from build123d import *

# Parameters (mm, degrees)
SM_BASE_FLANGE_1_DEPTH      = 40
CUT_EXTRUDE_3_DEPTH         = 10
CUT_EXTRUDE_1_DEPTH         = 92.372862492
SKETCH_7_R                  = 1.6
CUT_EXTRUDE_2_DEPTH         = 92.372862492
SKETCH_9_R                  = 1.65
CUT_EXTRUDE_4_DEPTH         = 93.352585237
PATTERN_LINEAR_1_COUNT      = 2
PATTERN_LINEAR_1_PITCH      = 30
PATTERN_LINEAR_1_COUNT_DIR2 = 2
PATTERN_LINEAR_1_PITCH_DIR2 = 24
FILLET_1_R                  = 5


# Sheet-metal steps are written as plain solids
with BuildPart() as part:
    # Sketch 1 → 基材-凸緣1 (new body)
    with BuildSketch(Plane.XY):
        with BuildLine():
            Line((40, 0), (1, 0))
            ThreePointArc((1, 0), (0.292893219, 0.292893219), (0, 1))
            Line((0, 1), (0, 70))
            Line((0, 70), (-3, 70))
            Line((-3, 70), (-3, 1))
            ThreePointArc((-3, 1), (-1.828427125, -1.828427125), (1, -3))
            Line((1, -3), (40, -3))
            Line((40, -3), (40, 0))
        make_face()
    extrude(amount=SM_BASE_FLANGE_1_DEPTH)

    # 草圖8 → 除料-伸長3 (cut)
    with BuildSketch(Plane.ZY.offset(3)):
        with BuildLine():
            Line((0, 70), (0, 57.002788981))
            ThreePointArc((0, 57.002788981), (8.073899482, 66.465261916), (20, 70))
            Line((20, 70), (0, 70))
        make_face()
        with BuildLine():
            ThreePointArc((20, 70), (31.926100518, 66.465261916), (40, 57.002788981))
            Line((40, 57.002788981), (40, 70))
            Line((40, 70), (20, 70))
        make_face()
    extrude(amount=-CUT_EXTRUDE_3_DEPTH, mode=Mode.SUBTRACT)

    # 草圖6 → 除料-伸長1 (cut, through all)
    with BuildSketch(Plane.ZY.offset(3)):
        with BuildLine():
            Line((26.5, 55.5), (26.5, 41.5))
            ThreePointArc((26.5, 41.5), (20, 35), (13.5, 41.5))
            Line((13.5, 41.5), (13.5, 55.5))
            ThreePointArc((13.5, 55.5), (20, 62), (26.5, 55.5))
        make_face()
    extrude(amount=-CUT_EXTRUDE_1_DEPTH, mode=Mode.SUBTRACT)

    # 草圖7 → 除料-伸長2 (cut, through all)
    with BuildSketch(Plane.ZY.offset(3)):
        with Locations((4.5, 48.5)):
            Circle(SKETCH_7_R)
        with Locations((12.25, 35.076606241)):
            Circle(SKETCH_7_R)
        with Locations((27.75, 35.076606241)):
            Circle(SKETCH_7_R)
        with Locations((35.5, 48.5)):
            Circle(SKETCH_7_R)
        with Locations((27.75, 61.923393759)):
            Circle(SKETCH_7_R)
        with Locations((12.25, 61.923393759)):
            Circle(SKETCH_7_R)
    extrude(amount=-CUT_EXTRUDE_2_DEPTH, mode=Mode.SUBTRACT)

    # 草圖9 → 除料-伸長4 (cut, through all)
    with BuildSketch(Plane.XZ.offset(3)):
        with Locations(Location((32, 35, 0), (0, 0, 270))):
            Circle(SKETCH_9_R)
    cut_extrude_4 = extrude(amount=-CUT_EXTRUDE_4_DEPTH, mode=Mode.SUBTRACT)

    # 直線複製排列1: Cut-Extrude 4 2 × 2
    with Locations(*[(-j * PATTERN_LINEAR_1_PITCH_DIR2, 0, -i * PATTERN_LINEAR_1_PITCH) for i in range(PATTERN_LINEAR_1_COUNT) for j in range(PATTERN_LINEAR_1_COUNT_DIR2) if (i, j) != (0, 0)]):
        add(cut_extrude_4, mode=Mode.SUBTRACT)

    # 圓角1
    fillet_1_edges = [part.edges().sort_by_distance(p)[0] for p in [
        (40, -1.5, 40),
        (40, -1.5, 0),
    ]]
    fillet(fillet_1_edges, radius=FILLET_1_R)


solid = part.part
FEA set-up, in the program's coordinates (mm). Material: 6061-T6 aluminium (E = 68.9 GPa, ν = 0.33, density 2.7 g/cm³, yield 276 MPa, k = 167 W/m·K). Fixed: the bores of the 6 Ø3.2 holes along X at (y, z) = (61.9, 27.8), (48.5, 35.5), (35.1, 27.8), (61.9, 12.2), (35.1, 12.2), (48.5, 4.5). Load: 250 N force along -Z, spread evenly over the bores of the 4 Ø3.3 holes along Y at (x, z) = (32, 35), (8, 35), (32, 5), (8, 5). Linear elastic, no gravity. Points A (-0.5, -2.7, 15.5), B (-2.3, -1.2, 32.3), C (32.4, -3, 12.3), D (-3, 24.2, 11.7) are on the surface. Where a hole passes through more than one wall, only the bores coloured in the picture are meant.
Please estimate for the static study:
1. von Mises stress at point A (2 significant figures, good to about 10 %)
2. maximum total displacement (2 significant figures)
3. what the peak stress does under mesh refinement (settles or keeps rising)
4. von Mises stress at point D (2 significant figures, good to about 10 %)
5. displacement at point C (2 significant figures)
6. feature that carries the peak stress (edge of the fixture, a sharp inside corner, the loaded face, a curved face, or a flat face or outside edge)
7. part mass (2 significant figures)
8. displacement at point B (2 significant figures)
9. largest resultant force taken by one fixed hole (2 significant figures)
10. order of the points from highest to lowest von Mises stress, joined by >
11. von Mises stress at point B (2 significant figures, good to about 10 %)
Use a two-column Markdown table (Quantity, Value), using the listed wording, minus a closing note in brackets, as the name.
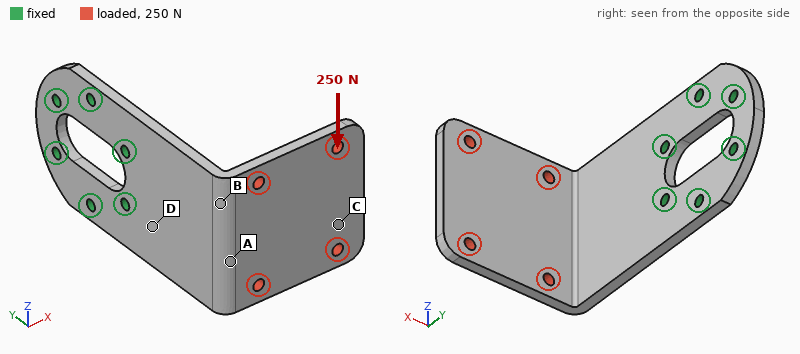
| Quantity | Value |
|---|---|
| von Mises stress at point A | 32 MPa |
| maximum total displacement | 0.68 mm |
| what the peak stress does under mesh refinement | keeps rising |
| von Mises stress at point D | 55 MPa |
| displacement at point C | 0.53 mm |
| feature that carries the peak stress | edge of the fixture |
| part mass | 32 g |
| displacement at point B | 0.18 mm |
| largest resultant force taken by one fixed hole | 380 N |
| order of the points from highest to lowest von Mises stress, joined by > | D > B > A > C |
| von Mises stress at point B | 41 MPa |
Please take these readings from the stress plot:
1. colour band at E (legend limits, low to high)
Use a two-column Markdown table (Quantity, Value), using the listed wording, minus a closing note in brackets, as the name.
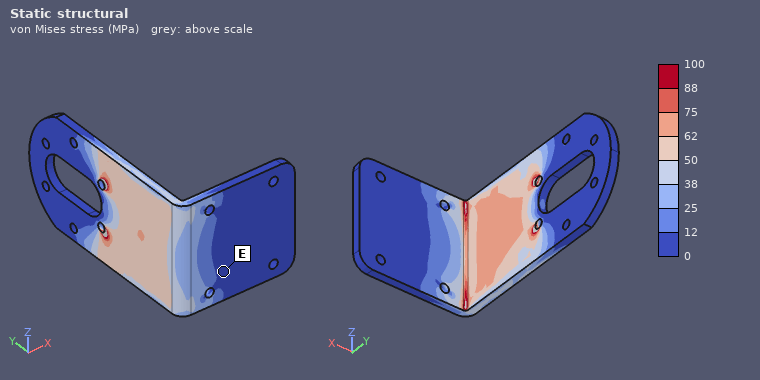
| Quantity | Value |
|---|---|
| colour band at E | 0 to 12 MPa |
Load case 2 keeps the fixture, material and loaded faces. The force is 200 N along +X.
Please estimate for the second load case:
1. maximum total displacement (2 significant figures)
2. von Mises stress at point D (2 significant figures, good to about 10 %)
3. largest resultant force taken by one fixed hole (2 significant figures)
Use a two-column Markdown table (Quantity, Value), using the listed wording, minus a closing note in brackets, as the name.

| Quantity | Value |
|---|---|
| maximum total displacement | 1.0 mm |
| von Mises stress at point D | 76 MPa |
| largest resultant force taken by one fixed hole | 190 N |
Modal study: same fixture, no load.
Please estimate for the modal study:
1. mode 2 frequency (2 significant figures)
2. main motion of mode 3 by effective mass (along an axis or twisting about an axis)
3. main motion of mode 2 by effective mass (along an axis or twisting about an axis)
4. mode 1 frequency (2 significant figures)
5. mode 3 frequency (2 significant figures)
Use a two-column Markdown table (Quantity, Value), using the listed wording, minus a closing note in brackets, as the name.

| Quantity | Value |
|---|---|
| mode 2 frequency | 960 Hz |
| main motion of mode 3 by effective mass | along X |
| main motion of mode 2 by effective mass | along Z |
| mode 1 frequency | 560 Hz |
| mode 3 frequency | 1500 Hz |
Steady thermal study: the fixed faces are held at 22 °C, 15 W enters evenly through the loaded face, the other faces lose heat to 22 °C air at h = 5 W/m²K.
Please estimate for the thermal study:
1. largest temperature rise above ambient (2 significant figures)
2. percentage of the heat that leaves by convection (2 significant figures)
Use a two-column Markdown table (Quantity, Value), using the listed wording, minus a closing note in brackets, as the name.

| Quantity | Value |
|---|---|
| largest temperature rise above ambient | 44 K |
| percentage of the heat that leaves by convection | 5.9 % |
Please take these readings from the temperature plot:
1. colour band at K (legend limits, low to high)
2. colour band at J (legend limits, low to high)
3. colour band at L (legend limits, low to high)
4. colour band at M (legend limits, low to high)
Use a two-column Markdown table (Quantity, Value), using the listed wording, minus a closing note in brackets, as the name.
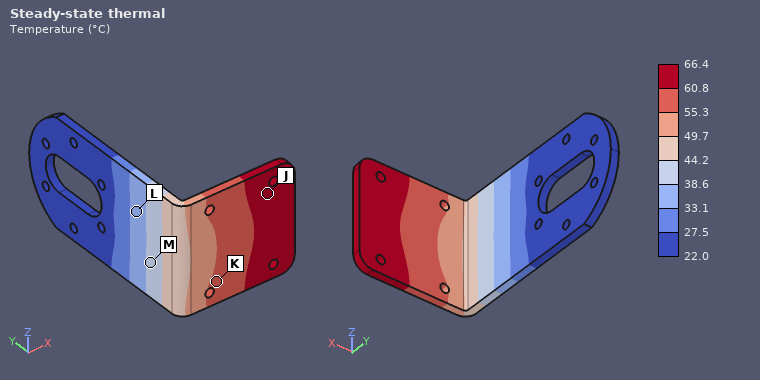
| Quantity | Value |
|---|---|
| colour band at K | 55.3 to 60.8 °C |
| colour band at J | 60.8 to 66.4 °C |
| colour band at L | 33.1 to 38.6 °C |
| colour band at M | 38.6 to 44.2 °C |
